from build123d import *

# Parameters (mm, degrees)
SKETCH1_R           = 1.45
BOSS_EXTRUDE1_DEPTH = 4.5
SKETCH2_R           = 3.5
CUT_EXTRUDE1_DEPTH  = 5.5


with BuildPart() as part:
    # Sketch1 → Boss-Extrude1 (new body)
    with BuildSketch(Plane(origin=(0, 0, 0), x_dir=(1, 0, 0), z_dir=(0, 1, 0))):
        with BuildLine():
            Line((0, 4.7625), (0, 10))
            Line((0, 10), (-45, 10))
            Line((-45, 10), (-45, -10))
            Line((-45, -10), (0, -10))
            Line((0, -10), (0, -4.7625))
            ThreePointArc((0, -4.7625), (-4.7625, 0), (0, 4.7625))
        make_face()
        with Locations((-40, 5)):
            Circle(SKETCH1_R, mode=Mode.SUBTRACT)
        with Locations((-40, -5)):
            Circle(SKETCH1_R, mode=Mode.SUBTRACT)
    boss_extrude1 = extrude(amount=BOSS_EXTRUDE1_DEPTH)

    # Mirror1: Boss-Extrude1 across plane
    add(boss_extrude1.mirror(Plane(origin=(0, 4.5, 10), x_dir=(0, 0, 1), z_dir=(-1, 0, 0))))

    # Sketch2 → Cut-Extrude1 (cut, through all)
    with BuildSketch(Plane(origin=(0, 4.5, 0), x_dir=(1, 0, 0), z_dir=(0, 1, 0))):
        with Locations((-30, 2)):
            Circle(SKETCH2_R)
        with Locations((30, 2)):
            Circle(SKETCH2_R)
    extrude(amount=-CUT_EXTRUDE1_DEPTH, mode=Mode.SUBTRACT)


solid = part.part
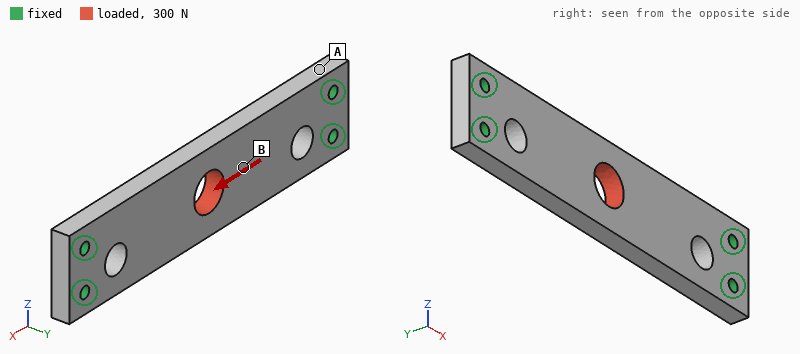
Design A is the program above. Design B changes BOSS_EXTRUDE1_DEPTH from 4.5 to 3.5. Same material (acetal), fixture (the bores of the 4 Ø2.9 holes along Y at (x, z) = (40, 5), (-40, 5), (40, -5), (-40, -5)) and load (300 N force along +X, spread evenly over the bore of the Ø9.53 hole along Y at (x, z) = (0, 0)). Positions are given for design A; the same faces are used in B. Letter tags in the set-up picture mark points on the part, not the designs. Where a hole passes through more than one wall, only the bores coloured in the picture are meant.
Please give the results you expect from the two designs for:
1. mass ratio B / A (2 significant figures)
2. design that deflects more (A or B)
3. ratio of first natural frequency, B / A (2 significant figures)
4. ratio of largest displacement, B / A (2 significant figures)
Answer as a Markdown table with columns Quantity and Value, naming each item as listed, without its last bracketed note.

| Quantity | Value |
|---|---|
| mass ratio B / A | 0.78 |
| design that deflects more | B |
| ratio of first natural frequency, B / A | 0.79 |
| ratio of largest displacement, B / A | 1.3 |
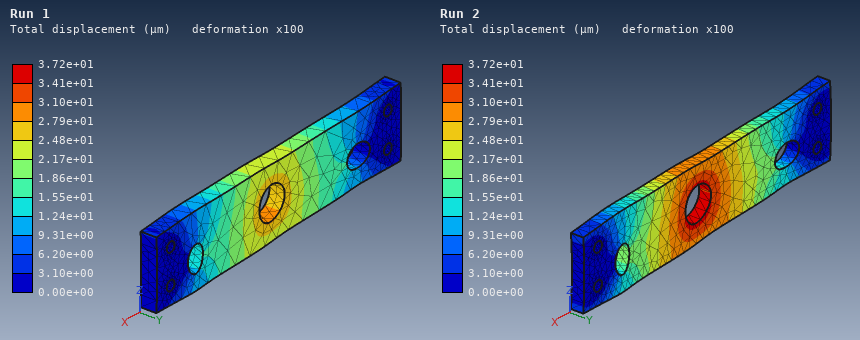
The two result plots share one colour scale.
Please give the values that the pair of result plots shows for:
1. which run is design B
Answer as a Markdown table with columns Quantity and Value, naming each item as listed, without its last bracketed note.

| Quantity | Value |
|---|---|
| which run is design B | Run 2 |
